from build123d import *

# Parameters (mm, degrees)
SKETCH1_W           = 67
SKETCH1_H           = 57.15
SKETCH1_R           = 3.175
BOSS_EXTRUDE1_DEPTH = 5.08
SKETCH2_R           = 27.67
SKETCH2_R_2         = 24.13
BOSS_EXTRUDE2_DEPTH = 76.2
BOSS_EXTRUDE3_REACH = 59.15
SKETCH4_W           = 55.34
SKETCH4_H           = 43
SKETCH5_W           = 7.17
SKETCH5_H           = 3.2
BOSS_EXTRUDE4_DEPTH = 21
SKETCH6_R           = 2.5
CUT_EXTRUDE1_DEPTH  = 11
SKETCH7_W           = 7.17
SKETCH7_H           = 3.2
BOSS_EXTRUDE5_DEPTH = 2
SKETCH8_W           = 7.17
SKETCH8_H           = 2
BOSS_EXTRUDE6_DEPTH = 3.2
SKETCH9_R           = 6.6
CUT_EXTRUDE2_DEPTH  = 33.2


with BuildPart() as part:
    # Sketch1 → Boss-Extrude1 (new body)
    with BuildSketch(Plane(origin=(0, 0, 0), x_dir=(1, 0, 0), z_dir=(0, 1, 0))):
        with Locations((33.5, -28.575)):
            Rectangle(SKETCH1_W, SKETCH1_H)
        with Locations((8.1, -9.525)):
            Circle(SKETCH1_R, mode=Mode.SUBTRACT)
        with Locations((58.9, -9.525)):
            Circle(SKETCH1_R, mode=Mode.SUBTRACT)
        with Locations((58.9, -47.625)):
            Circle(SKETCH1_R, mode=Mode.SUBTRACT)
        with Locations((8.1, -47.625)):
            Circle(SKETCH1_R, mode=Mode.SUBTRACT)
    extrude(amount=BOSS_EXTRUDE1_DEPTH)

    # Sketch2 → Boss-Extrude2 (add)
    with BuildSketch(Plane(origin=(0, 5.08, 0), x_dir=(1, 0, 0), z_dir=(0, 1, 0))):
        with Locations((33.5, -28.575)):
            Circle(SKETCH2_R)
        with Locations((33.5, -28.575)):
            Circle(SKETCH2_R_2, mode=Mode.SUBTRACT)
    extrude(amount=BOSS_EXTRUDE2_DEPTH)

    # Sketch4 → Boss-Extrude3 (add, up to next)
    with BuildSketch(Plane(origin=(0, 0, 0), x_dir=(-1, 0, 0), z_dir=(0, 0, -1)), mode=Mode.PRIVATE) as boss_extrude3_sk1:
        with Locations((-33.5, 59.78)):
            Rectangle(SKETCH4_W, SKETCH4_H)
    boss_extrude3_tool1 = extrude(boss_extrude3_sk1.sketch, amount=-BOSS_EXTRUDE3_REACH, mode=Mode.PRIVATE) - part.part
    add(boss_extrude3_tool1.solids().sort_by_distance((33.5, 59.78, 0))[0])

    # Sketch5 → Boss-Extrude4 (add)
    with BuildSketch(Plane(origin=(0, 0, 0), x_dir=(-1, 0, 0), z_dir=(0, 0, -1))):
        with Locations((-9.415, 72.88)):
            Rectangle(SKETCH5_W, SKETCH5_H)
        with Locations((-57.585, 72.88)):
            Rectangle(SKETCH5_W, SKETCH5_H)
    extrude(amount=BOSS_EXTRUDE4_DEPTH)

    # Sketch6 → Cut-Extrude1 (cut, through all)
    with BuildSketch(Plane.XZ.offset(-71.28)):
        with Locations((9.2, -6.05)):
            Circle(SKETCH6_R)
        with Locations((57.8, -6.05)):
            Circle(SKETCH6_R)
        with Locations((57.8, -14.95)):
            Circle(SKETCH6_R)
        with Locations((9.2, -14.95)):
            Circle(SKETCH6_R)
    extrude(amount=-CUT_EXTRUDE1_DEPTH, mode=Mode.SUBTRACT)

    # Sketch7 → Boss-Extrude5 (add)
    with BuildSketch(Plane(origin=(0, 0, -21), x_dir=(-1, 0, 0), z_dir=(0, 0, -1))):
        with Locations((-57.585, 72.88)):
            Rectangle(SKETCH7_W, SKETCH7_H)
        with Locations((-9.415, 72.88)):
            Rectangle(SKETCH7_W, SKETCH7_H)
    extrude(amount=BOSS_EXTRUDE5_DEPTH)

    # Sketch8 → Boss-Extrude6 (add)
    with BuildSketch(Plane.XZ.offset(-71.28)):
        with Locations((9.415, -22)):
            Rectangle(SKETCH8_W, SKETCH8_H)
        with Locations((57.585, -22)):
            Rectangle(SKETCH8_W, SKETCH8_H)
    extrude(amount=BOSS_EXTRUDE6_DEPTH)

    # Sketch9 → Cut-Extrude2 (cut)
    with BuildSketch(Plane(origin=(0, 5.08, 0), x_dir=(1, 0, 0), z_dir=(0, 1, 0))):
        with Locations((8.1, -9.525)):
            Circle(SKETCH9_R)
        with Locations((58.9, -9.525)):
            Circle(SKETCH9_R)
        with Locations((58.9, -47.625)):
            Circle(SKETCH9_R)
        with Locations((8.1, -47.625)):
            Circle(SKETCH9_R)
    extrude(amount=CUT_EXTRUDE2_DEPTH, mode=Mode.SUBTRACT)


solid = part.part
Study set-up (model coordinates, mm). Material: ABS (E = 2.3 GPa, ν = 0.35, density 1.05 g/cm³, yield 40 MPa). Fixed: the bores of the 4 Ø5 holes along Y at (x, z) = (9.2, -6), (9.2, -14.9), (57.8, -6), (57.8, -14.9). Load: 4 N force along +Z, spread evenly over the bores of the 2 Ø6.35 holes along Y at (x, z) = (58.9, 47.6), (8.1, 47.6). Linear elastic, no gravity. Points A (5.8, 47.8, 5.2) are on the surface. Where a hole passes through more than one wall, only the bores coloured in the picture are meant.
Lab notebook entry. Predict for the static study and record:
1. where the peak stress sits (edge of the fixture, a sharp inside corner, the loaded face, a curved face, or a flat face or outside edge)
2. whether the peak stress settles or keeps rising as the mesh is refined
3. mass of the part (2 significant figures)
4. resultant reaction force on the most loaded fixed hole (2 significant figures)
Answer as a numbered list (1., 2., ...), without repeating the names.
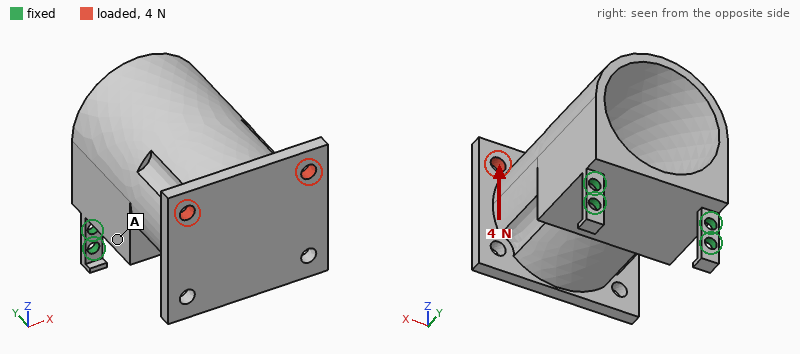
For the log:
1. edge of the fixture
2. keeps rising
3. 82 g
4. 2.1 N
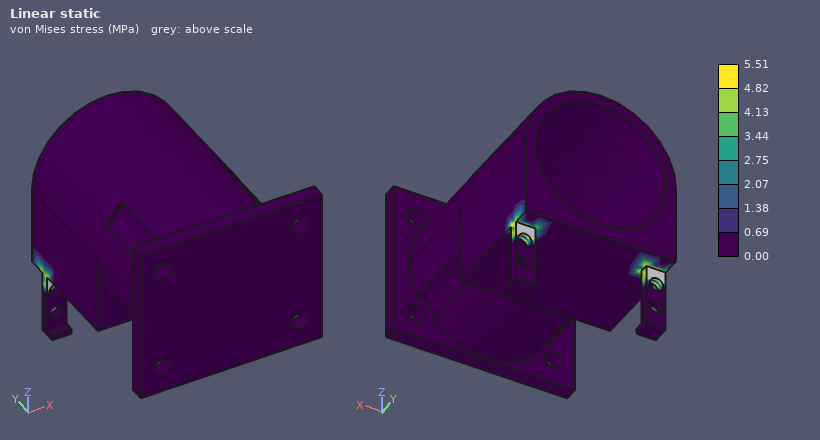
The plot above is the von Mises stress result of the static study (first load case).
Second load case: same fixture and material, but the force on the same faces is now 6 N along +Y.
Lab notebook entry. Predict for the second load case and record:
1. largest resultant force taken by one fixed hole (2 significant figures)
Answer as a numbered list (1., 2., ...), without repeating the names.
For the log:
1. 3.1 N
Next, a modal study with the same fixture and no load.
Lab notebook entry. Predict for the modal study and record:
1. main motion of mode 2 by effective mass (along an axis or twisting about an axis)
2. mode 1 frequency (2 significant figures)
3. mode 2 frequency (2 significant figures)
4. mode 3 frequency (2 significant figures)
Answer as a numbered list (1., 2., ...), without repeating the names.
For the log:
1. along X
2. 45 Hz
3. 420 Hz
4. 640 Hz
